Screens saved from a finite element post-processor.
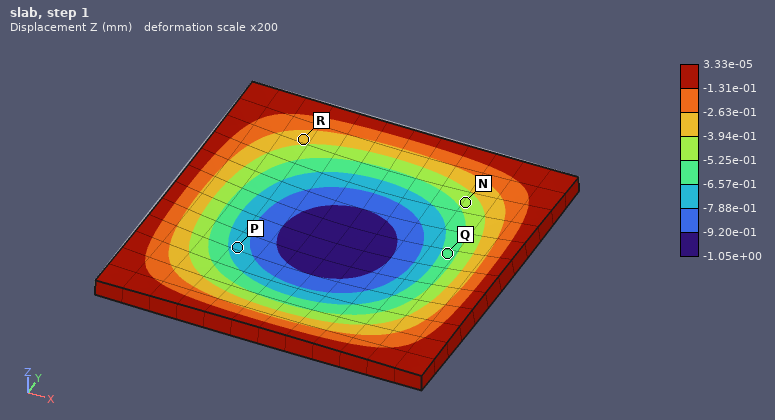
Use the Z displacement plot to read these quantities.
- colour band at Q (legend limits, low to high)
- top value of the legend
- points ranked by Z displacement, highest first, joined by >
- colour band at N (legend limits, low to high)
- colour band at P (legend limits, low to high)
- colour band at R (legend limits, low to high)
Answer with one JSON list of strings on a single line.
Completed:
["-6.57e-01 to -5.25e-01 mm", "3.33e-05 mm", "R > N > Q > P", "-5.25e-01 to -3.94e-01 mm", "-7.88e-01 to -6.57e-01 mm", "-3.94e-01 to -2.63e-01 mm"]
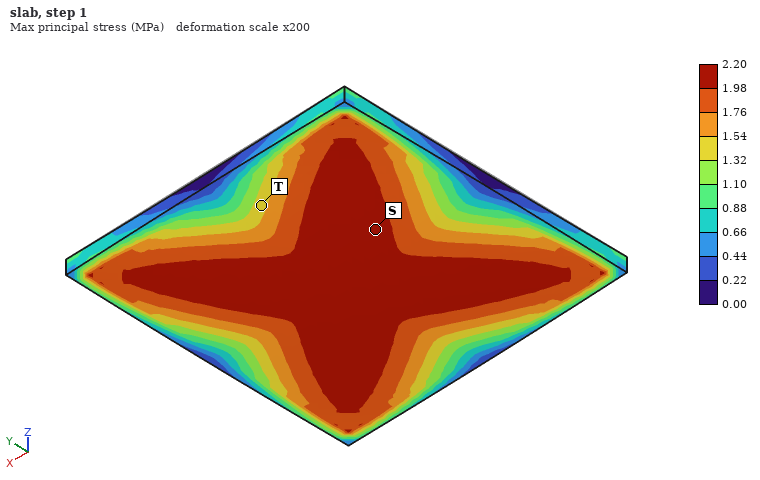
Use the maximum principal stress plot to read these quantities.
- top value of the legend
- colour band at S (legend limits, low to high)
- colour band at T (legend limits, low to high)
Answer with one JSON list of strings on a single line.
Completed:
["2.20 MPa", "1.98 to 2.20 MPa", "1.32 to 1.54 MPa"]
